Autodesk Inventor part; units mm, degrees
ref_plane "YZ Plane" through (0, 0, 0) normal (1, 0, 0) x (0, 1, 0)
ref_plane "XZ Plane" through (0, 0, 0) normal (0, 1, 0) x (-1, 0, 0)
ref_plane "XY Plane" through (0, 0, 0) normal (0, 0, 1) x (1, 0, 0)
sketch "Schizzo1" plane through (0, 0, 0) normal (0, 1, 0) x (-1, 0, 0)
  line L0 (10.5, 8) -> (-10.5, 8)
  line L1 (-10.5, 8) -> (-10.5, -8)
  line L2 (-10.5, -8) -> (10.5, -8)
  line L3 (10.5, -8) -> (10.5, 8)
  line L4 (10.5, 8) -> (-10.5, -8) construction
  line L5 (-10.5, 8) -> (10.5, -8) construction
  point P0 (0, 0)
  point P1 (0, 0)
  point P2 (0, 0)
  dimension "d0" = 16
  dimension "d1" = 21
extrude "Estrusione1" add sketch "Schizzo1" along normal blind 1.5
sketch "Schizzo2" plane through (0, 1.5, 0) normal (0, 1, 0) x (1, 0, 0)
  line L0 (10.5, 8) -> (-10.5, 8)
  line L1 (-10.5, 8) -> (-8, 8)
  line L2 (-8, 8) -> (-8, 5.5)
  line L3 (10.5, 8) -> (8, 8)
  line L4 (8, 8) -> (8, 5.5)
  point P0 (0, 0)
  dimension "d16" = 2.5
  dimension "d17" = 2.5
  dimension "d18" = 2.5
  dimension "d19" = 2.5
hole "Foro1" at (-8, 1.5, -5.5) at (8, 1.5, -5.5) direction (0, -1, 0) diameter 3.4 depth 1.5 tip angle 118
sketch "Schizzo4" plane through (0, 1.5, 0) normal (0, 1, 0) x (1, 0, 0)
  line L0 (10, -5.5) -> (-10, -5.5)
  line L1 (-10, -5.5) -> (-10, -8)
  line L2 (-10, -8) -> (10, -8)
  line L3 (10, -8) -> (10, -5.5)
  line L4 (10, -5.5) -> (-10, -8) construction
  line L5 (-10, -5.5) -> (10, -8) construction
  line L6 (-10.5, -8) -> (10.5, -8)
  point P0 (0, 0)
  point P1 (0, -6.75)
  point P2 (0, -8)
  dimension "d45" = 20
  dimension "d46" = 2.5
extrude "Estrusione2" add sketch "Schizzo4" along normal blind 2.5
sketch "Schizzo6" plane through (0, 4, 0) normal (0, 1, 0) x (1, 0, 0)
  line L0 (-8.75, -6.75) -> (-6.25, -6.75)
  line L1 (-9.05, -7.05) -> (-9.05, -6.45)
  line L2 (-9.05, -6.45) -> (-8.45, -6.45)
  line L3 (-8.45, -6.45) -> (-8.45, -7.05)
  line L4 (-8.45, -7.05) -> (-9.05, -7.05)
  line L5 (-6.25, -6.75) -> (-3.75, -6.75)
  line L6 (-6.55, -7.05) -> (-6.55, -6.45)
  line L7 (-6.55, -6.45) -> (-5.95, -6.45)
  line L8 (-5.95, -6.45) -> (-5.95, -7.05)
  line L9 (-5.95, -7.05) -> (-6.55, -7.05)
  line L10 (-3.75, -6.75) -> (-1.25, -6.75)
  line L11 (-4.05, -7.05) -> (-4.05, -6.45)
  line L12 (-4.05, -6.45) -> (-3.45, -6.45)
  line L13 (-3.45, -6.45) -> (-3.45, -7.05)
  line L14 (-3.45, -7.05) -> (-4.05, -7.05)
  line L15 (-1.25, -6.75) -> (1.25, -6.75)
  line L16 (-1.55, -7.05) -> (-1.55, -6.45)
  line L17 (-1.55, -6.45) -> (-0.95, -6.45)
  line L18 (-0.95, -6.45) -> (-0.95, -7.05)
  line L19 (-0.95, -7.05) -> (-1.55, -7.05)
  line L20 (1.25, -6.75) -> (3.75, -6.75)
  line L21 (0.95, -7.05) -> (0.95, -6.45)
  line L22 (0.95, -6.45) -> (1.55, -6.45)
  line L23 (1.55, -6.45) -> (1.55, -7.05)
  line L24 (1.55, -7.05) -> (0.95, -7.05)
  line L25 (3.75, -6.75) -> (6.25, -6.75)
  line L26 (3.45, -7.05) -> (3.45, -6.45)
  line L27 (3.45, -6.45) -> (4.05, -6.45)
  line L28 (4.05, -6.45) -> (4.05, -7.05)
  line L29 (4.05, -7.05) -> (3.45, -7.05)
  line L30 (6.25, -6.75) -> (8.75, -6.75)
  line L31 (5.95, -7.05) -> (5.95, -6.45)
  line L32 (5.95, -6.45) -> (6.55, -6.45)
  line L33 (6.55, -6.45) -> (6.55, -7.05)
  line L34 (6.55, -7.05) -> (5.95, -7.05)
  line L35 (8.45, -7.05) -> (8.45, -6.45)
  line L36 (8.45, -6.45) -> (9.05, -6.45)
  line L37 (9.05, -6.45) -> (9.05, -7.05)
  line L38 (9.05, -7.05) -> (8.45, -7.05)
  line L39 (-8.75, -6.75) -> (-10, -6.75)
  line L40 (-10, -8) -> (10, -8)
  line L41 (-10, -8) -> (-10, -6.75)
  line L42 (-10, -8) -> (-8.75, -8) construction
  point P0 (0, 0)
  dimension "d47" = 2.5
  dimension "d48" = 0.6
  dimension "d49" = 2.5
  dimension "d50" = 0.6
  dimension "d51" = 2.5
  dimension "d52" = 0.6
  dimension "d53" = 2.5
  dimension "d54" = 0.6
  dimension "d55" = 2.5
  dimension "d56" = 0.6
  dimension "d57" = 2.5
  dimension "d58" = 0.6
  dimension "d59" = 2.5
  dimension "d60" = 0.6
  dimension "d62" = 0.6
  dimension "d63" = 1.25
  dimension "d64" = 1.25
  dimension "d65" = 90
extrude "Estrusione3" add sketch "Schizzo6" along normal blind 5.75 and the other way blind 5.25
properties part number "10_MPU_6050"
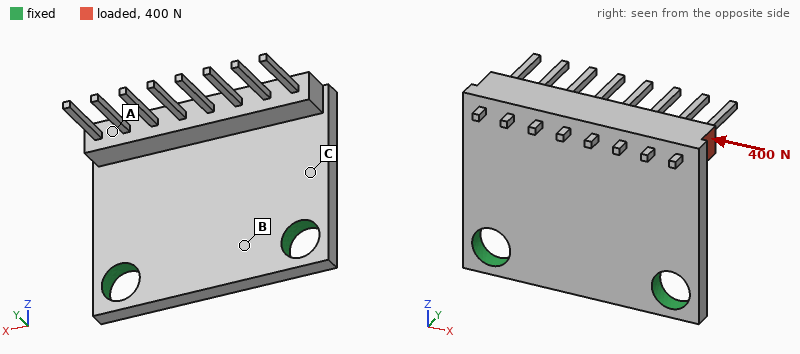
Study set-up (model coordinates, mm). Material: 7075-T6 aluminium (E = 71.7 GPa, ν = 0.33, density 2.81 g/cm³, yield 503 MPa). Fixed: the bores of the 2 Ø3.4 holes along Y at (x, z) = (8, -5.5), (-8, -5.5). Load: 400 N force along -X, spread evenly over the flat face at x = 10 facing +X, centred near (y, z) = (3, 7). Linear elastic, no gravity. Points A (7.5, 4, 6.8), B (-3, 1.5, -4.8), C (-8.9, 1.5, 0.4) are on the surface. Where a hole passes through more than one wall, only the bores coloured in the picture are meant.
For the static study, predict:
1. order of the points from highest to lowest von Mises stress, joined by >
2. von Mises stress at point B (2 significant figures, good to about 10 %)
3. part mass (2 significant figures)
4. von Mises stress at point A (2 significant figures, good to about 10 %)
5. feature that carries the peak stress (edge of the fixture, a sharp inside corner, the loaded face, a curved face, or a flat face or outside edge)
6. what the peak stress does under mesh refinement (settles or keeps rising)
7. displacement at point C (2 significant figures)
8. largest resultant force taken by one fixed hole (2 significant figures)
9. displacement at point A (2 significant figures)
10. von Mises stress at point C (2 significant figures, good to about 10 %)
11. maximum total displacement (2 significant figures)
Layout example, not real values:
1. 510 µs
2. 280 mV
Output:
1. A > C > B
2. 20 MPa
3. 1.7 g
4. 78 MPa
5. edge of the fixture
6. keeps rising
7. 15 µm
8. 350 N
9. 47 µm
10. 44 MPa
11. 85 µm
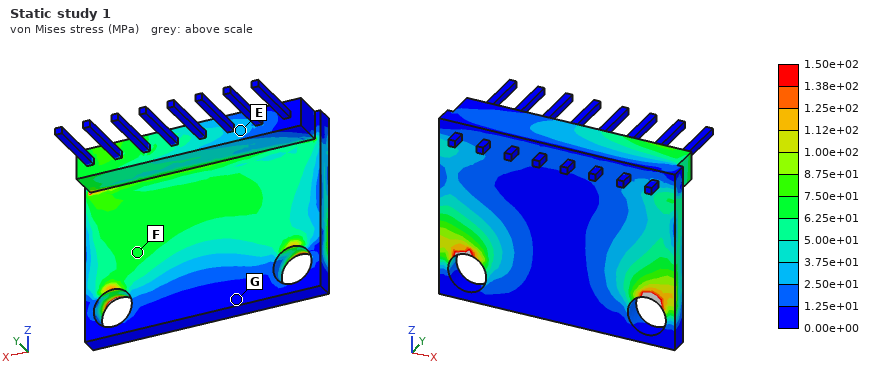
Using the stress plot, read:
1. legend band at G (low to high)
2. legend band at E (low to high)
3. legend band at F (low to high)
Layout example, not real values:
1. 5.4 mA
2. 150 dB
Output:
1. 0.00e+00 to 1.25e+01 MPa
2. 2.50e+01 to 3.75e+01 MPa
3. 6.25e+01 to 7.50e+01 MPa
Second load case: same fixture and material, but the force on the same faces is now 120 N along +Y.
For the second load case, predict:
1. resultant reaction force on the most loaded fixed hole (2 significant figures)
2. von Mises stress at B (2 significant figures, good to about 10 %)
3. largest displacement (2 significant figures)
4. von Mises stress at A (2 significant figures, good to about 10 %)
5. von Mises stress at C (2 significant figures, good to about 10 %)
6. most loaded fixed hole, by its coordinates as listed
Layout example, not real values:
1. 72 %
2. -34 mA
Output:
1. 130 N
2. 60 MPa
3. 0.31 mm
4. 47 MPa
5. 90 MPa
6. (8, -5.5)
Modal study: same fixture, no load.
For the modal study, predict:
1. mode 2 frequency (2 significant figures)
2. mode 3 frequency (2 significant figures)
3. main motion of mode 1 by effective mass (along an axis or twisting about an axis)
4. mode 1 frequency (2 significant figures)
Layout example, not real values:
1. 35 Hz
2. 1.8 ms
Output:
1. 11 kHz
2. 14 kHz
3. along Y
4. 4900 Hz
